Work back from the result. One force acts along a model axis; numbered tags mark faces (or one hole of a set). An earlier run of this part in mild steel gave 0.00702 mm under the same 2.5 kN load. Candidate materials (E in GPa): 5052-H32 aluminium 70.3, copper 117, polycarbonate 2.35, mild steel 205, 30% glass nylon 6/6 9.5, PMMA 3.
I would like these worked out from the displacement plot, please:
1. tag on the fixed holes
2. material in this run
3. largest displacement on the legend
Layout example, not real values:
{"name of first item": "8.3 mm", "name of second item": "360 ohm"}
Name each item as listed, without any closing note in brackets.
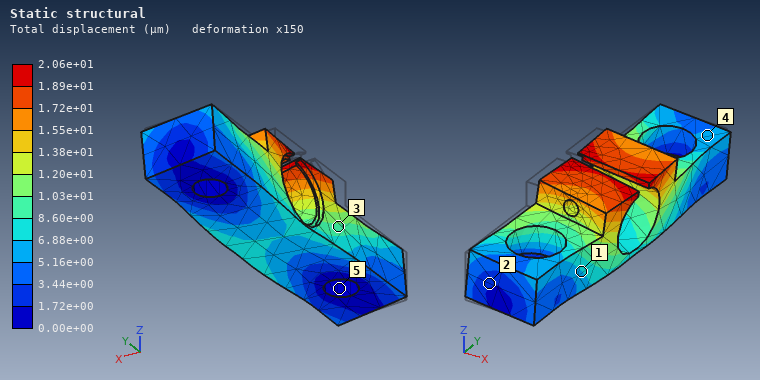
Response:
{"tag on the fixed holes": "5", "material in this run": "5052-H32 aluminium", "largest displacement on the legend": "2.06e+01 µm"}
